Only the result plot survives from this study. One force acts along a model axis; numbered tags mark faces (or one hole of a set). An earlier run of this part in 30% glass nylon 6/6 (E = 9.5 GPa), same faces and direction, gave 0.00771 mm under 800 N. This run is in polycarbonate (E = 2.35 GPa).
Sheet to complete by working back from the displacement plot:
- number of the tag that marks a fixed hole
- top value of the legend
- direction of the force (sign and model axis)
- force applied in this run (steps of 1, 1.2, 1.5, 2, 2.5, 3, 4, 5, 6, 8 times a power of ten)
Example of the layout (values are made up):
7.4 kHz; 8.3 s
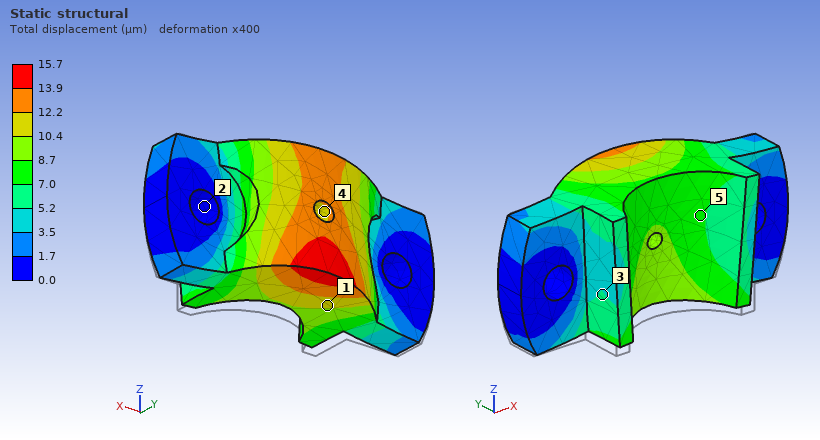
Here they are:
2; 15.7 µm; +Z; 400 N
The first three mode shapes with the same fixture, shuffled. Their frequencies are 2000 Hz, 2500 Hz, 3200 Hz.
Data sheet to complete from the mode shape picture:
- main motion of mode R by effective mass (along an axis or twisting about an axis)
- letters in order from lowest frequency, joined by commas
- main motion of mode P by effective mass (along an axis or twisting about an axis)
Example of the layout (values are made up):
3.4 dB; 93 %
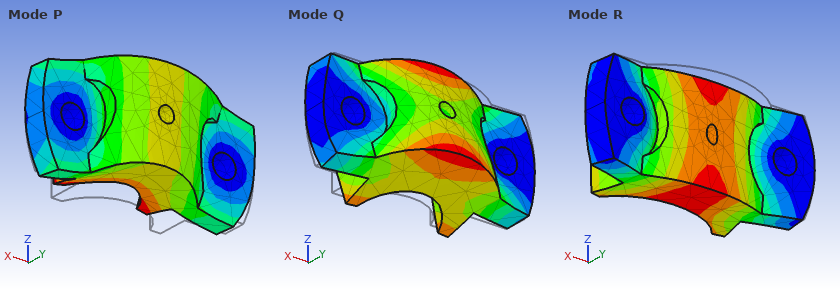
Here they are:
along Y; Q, R, P; along Z
